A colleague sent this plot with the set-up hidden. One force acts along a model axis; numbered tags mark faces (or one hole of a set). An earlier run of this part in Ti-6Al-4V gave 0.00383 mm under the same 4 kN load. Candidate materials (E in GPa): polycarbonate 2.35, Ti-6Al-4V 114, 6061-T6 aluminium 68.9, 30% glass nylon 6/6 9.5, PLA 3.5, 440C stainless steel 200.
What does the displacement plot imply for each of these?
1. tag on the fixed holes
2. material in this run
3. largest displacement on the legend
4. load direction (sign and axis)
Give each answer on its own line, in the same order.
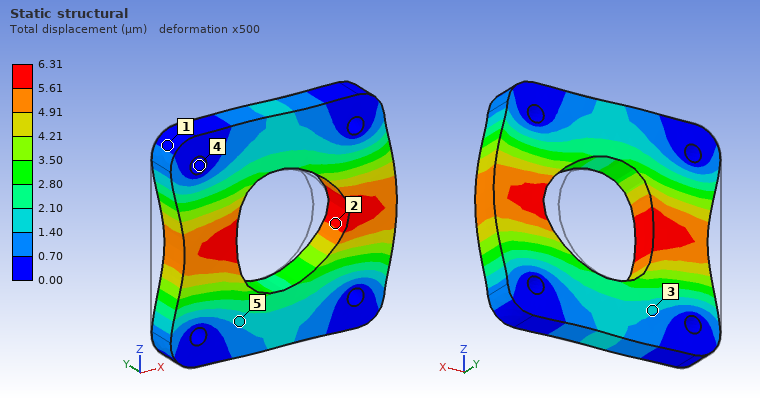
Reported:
4
6061-T6 aluminium
6.31 µm
+X
